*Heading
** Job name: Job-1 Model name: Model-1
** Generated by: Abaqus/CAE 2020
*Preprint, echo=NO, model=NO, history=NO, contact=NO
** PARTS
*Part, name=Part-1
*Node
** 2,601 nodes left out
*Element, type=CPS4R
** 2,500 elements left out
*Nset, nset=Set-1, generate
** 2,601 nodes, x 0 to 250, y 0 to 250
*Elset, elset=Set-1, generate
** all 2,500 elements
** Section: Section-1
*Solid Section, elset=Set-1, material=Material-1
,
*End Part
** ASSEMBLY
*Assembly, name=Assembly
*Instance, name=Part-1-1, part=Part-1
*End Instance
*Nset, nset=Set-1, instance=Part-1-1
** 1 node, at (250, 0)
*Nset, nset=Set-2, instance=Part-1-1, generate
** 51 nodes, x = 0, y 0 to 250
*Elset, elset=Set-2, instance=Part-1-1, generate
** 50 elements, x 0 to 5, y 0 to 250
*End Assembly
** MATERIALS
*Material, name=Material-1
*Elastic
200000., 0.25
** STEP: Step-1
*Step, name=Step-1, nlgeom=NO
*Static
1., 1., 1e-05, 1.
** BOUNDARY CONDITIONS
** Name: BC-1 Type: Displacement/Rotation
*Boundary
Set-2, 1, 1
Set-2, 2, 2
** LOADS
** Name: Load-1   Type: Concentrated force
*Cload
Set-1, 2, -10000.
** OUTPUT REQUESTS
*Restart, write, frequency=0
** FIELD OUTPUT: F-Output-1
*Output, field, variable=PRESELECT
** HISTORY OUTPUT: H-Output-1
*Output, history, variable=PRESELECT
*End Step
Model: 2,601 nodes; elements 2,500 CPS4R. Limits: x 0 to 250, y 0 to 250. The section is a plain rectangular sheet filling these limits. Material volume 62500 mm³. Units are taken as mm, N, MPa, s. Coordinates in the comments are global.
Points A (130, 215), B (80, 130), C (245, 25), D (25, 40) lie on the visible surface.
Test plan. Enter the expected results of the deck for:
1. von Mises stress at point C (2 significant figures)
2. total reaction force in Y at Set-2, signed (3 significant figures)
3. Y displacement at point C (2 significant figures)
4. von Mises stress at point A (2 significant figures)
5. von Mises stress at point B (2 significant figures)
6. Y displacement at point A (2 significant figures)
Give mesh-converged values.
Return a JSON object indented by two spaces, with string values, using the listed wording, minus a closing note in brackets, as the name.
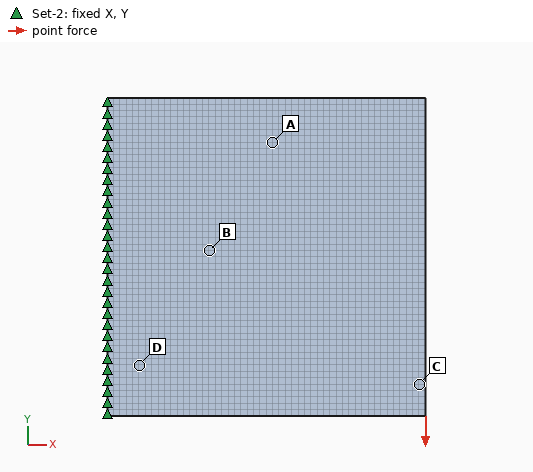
{
  "von Mises stress at point C": "720 MPa",
  "total reaction force in Y at Set-2, signed": "10000 N",
  "Y displacement at point C": "-0.47 mm",
  "von Mises stress at point A": "94 MPa",
  "von Mises stress at point B": "110 MPa",
  "Y displacement at point A": "-0.14 mm"
}
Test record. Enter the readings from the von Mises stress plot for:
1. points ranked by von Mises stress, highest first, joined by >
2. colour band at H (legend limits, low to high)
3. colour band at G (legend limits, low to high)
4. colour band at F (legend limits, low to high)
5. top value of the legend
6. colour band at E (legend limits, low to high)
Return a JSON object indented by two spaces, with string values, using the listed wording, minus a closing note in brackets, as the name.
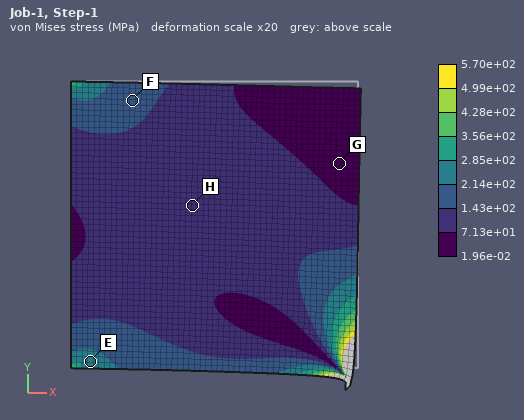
{
  "points ranked by von Mises stress, highest first, joined by >": "E > F > H > G",
  "colour band at H": "7.13e+01 to 1.43e+02 MPa",
  "colour band at G": "1.96e-02 to 7.13e+01 MPa",
  "colour band at F": "1.43e+02 to 2.14e+02 MPa",
  "top value of the legend": "5.70e+02 MPa",
  "colour band at E": "2.14e+02 to 2.85e+02 MPa"
}
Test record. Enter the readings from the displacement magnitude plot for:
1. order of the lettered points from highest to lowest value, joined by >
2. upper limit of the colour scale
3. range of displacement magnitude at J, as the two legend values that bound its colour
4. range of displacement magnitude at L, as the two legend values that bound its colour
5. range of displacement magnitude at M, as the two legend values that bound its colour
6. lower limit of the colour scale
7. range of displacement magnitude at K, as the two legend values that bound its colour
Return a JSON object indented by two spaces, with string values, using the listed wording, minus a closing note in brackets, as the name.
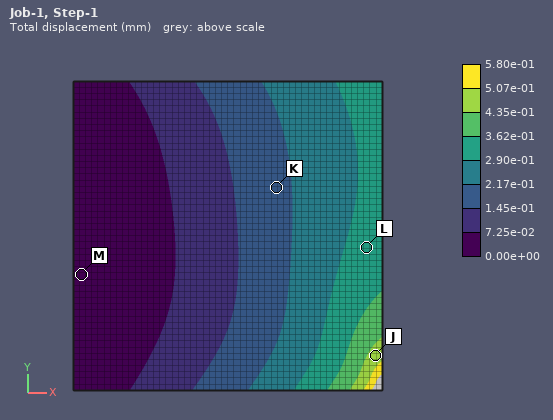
{
  "order of the lettered points from highest to lowest value, joined by >": "J > L > K > M",
  "upper limit of the colour scale": "5.80e-01 mm",
  "range of displacement magnitude at J, as the two legend values that bound its colour": "4.35e-01 to 5.07e-01 mm",
  "range of displacement magnitude at L, as the two legend values that bound its colour": "2.90e-01 to 3.62e-01 mm",
  "range of displacement magnitude at M, as the two legend values that bound its colour": "0.00e+00 to 7.25e-02 mm",
  "lower limit of the colour scale": "0.00e+00 mm",
  "range of displacement magnitude at K, as the two legend values that bound its colour": "1.45e-01 to 2.17e-01 mm"
}
